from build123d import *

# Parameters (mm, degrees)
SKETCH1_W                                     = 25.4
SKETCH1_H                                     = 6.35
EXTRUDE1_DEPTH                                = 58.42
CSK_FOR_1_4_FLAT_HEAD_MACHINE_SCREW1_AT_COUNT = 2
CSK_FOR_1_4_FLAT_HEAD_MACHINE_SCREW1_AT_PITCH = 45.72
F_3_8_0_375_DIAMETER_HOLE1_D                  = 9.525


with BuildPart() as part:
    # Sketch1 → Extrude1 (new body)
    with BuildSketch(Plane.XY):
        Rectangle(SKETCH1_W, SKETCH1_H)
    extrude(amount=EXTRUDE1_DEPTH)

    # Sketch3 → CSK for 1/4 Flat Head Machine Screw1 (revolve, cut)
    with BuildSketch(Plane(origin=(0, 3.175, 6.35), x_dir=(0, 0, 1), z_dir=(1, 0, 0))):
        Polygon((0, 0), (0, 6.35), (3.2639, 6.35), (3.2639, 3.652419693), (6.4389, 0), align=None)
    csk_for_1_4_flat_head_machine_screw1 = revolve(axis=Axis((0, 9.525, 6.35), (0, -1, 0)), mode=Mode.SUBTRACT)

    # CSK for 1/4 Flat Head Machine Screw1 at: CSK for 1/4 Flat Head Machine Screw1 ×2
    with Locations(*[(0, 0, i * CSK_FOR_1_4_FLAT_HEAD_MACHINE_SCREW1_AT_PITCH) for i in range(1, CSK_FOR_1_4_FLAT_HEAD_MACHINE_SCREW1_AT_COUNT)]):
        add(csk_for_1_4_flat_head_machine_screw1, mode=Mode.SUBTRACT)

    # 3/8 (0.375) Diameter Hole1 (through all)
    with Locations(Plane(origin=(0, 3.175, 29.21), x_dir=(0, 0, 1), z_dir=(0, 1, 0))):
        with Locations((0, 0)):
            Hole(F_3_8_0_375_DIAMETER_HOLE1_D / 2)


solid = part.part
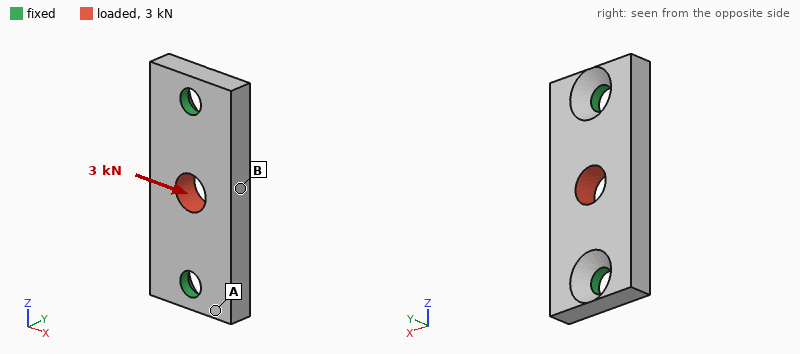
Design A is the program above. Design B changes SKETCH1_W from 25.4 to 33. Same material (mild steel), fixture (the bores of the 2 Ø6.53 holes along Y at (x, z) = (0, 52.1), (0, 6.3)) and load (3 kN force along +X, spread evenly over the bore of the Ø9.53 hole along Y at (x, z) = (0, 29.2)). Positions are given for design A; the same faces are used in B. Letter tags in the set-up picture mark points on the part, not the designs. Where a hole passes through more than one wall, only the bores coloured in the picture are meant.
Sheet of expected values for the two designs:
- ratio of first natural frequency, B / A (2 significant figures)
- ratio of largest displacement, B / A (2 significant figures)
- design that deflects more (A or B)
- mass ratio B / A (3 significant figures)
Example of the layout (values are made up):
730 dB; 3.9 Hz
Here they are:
0.69; 0.89; A; 1.34
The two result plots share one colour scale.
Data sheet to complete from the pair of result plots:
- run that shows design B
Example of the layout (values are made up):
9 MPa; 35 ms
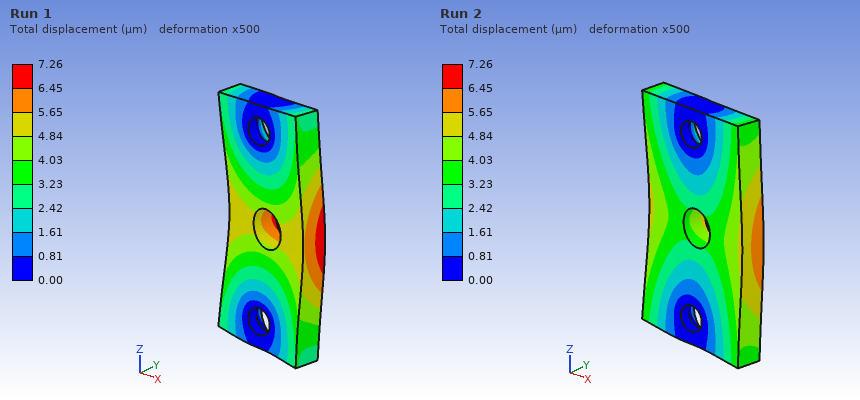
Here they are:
Run 2
